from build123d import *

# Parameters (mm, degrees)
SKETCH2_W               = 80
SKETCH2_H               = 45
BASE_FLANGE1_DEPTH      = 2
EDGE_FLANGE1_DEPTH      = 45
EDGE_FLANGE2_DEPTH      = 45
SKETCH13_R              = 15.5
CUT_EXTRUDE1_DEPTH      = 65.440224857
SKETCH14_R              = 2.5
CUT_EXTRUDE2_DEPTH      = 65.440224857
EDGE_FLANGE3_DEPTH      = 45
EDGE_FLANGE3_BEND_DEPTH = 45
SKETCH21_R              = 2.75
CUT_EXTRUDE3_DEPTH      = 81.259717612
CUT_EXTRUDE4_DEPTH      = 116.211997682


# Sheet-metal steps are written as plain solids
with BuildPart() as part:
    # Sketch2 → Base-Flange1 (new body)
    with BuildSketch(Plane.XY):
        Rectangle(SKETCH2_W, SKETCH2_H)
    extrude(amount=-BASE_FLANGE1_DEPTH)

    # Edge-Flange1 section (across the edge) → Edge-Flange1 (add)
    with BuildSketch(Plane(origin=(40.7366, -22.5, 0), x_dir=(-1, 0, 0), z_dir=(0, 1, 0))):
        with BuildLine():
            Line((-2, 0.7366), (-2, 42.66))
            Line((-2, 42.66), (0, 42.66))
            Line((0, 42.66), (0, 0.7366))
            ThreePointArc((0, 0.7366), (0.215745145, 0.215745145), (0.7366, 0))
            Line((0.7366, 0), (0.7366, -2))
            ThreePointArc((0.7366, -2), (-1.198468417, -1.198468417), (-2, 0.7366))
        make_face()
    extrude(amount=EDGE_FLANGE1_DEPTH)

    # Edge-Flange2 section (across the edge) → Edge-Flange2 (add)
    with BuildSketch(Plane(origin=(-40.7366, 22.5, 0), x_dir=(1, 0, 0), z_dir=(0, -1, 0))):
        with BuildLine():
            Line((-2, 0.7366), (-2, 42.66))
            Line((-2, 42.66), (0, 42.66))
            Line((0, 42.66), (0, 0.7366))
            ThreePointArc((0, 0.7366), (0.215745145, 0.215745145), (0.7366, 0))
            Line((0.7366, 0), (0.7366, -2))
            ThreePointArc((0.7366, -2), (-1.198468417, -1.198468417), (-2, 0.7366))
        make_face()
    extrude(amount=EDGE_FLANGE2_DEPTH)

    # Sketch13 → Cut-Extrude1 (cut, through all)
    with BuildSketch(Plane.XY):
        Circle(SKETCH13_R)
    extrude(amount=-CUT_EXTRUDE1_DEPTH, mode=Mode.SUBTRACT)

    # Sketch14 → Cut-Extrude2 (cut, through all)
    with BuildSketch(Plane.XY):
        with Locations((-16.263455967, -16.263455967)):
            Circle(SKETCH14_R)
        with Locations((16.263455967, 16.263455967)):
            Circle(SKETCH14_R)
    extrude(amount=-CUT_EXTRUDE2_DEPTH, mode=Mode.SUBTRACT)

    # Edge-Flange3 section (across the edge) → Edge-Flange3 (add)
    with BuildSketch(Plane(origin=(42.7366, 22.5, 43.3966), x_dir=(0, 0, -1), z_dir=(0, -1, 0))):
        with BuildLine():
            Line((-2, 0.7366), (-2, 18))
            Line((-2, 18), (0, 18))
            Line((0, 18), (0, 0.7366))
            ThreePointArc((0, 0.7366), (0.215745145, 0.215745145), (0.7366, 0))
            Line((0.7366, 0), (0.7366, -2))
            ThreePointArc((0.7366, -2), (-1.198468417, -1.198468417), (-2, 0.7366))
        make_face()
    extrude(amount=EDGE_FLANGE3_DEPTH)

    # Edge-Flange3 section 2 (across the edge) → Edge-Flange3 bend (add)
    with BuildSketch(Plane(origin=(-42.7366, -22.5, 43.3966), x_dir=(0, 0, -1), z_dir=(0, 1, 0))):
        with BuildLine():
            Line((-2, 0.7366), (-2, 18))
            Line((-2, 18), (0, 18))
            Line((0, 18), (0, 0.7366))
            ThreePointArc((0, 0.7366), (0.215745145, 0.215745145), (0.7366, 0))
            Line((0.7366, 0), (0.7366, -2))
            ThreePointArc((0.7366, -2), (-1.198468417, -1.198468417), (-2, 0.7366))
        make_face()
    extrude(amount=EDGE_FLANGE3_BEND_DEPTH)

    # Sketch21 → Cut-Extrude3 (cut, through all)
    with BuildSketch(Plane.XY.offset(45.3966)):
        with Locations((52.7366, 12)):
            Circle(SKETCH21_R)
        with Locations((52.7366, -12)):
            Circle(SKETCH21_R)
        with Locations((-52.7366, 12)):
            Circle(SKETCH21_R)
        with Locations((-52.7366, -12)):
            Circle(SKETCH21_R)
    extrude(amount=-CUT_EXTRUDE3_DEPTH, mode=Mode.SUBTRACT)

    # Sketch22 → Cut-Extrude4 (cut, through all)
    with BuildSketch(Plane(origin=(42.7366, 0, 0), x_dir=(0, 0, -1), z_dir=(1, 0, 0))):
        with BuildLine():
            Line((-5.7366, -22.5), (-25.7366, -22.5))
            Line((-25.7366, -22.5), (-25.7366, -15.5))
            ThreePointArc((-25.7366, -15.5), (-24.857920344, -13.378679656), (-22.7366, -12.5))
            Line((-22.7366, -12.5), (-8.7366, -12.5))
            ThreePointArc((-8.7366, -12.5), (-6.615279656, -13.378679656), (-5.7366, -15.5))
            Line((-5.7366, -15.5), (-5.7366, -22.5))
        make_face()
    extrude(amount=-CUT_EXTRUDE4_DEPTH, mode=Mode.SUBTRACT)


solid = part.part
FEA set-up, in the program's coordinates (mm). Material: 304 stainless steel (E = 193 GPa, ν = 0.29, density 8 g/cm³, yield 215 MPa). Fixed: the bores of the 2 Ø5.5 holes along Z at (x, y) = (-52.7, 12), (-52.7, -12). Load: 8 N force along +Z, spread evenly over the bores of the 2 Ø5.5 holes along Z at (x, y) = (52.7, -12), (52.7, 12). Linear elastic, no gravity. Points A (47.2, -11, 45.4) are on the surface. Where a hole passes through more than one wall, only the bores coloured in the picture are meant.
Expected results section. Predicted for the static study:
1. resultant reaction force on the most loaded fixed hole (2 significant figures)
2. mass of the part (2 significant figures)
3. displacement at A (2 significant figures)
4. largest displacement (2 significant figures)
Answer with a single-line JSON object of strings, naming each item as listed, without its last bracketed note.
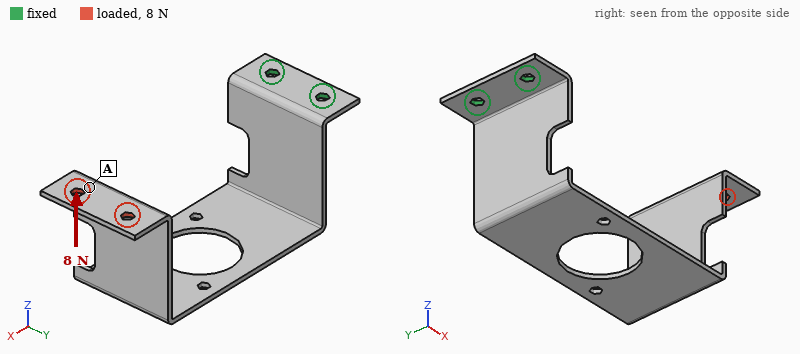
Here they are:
{"resultant reaction force on the most loaded fixed hole": "5.6 N", "mass of the part": "130 g", "displacement at A": "1.4 mm", "largest displacement": "1.6 mm"}
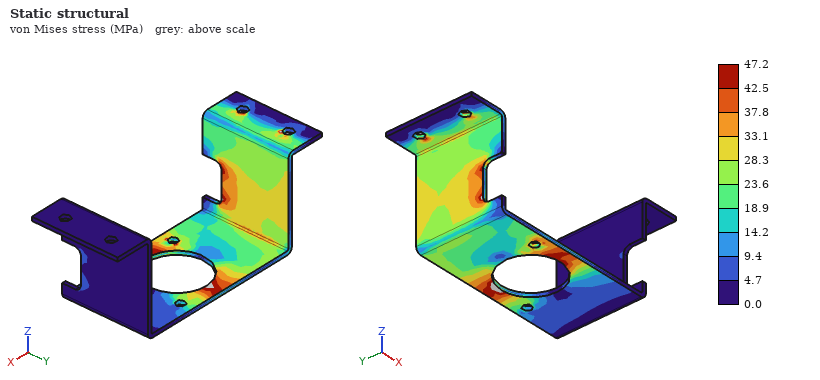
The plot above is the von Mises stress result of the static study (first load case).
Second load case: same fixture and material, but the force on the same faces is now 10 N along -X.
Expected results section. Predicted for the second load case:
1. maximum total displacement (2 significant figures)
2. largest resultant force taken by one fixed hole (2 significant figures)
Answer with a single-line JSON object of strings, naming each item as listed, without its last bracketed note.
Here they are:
{"maximum total displacement": "1.1 mm", "largest resultant force taken by one fixed hole": "5.0 N"}
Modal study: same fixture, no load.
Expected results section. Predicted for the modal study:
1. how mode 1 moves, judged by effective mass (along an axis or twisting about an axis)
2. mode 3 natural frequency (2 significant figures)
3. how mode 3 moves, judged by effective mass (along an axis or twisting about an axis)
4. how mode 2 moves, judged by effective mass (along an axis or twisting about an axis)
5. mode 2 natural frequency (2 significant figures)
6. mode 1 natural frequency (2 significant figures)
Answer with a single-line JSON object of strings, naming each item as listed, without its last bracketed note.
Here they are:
{"how mode 1 moves, judged by effective mass": "along Z", "mode 3 natural frequency": "160 Hz", "how mode 3 moves, judged by effective mass": "along X", "how mode 2 moves, judged by effective mass": "along Y", "mode 2 natural frequency": "98 Hz", "mode 1 natural frequency": "55 Hz"}
